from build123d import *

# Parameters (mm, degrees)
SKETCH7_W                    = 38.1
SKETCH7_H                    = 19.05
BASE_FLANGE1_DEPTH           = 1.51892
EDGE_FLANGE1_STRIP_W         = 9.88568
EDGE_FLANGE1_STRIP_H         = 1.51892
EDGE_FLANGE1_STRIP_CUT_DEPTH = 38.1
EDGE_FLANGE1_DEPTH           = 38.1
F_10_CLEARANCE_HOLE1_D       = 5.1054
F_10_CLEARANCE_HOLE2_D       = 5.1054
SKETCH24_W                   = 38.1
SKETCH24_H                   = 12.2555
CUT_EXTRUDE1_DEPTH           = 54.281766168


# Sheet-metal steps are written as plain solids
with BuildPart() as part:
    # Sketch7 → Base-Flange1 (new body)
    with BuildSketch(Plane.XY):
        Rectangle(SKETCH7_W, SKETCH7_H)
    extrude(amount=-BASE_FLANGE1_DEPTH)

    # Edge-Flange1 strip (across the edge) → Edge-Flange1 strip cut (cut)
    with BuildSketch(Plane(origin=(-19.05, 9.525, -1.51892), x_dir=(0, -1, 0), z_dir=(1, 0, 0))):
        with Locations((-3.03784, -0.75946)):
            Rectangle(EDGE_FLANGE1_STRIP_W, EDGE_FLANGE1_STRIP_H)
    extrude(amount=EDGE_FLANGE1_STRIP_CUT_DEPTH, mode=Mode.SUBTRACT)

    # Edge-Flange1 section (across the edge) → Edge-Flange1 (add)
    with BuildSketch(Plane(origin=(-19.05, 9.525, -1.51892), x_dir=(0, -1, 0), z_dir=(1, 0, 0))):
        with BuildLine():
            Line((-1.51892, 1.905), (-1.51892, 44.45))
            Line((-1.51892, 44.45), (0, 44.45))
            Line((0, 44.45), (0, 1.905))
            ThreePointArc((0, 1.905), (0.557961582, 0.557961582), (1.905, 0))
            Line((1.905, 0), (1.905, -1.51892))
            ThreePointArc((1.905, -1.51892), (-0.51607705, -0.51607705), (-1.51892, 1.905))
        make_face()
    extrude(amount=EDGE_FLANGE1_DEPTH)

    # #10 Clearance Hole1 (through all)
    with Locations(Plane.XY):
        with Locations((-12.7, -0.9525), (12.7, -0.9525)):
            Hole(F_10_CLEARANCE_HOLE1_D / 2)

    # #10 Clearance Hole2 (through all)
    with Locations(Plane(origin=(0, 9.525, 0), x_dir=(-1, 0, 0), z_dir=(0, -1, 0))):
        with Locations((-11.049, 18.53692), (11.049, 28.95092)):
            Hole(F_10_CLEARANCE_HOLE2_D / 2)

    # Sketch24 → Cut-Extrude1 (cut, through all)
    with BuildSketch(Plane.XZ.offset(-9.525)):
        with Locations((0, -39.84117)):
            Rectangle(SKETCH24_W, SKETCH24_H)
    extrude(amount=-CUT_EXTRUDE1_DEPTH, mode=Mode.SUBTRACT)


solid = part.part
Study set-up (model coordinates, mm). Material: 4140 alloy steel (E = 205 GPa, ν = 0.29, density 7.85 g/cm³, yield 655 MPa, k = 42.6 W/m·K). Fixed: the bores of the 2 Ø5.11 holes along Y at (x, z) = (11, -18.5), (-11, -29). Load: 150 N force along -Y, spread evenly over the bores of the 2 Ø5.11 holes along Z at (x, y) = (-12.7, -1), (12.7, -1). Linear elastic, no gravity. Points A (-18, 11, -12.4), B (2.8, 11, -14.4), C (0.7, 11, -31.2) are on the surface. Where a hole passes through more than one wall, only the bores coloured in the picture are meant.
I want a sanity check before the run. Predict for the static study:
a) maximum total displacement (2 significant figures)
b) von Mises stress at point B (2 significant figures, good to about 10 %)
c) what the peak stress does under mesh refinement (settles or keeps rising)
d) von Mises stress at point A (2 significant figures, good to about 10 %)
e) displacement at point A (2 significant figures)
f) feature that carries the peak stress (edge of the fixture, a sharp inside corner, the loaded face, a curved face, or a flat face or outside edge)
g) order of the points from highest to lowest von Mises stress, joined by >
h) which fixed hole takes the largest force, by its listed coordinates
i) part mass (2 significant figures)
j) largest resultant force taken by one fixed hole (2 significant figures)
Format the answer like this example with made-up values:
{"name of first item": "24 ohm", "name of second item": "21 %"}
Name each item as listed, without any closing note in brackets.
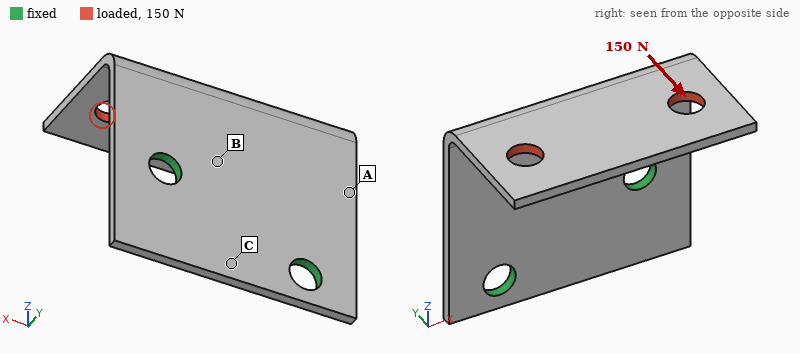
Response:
{"maximum total displacement": "0.36 mm", "von Mises stress at point B": "130 MPa", "what the peak stress does under mesh refinement": "keeps rising", "von Mises stress at point A": "80 MPa", "displacement at point A": "0.096 mm", "feature that carries the peak stress": "edge of the fixture", "order of the points from highest to lowest von Mises stress, joined by >": "B > A > C", "which fixed hole takes the largest force, by its listed coordinates": "(11, -18.5)", "part mass": "22 g", "largest resultant force taken by one fixed hole": "120 N"}
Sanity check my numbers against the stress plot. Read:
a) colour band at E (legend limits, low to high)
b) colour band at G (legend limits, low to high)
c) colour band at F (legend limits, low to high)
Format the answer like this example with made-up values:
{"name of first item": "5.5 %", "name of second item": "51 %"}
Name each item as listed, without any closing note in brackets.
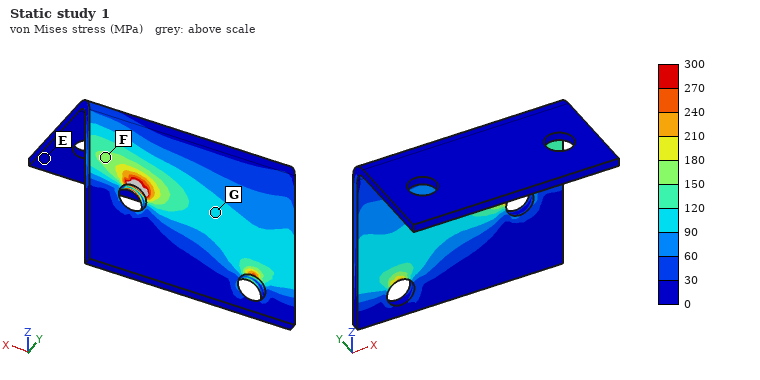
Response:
{"colour band at E": "0 to 30 MPa", "colour band at G": "90 to 120 MPa", "colour band at F": "150 to 180 MPa"}
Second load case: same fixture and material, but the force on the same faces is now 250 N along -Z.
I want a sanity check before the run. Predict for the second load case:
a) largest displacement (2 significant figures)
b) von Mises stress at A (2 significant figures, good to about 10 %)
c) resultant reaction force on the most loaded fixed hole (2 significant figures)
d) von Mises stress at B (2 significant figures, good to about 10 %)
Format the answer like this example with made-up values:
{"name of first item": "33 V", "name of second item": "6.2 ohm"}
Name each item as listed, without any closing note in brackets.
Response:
{"largest displacement": "0.62 mm", "von Mises stress at A": "150 MPa", "resultant reaction force on the most loaded fixed hole": "130 N", "von Mises stress at B": "170 MPa"}
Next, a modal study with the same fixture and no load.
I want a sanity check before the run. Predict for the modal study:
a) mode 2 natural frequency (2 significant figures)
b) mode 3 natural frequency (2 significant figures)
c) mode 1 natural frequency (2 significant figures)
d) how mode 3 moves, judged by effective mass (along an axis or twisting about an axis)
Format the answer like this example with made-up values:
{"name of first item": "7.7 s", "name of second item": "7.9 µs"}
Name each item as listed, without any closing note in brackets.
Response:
{"mode 2 natural frequency": "1900 Hz", "mode 3 natural frequency": "3200 Hz", "mode 1 natural frequency": "1100 Hz", "how mode 3 moves, judged by effective mass": "along Y"}
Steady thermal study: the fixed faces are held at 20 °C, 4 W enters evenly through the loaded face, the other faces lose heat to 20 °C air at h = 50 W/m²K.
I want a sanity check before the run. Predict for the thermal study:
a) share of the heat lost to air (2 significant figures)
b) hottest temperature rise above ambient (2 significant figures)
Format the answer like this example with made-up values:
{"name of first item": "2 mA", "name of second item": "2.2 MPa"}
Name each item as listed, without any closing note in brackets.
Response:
{"share of the heat lost to air": "61 %", "hottest temperature rise above ambient": "32 K"}
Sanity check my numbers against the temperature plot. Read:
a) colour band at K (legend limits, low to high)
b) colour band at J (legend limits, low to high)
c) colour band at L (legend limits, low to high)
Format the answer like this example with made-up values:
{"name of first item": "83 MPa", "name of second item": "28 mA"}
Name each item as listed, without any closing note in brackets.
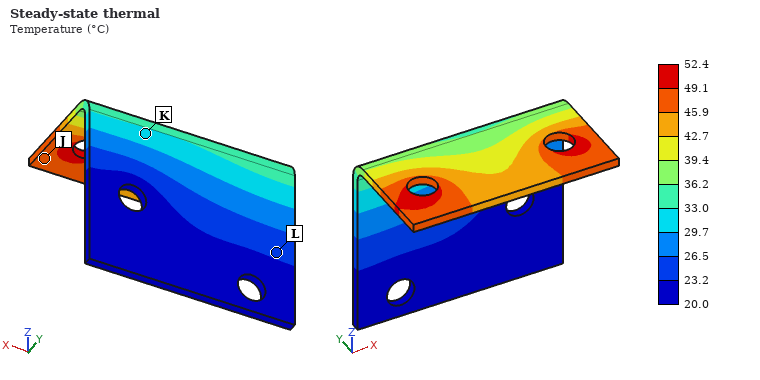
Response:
{"colour band at K": "29.7 to 33.0 °C", "colour band at J": "45.9 to 49.1 °C", "colour band at L": "23.2 to 26.5 °C"}
